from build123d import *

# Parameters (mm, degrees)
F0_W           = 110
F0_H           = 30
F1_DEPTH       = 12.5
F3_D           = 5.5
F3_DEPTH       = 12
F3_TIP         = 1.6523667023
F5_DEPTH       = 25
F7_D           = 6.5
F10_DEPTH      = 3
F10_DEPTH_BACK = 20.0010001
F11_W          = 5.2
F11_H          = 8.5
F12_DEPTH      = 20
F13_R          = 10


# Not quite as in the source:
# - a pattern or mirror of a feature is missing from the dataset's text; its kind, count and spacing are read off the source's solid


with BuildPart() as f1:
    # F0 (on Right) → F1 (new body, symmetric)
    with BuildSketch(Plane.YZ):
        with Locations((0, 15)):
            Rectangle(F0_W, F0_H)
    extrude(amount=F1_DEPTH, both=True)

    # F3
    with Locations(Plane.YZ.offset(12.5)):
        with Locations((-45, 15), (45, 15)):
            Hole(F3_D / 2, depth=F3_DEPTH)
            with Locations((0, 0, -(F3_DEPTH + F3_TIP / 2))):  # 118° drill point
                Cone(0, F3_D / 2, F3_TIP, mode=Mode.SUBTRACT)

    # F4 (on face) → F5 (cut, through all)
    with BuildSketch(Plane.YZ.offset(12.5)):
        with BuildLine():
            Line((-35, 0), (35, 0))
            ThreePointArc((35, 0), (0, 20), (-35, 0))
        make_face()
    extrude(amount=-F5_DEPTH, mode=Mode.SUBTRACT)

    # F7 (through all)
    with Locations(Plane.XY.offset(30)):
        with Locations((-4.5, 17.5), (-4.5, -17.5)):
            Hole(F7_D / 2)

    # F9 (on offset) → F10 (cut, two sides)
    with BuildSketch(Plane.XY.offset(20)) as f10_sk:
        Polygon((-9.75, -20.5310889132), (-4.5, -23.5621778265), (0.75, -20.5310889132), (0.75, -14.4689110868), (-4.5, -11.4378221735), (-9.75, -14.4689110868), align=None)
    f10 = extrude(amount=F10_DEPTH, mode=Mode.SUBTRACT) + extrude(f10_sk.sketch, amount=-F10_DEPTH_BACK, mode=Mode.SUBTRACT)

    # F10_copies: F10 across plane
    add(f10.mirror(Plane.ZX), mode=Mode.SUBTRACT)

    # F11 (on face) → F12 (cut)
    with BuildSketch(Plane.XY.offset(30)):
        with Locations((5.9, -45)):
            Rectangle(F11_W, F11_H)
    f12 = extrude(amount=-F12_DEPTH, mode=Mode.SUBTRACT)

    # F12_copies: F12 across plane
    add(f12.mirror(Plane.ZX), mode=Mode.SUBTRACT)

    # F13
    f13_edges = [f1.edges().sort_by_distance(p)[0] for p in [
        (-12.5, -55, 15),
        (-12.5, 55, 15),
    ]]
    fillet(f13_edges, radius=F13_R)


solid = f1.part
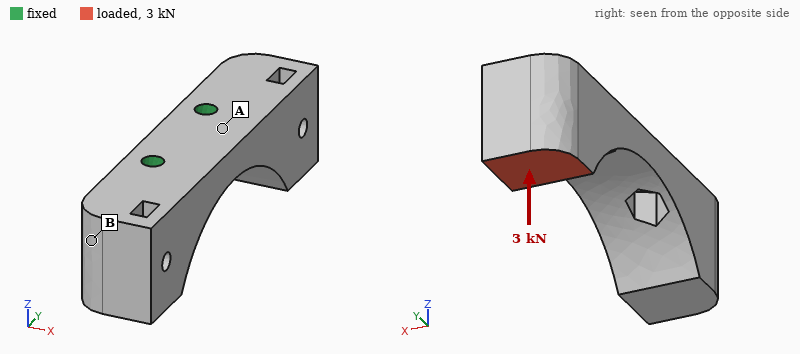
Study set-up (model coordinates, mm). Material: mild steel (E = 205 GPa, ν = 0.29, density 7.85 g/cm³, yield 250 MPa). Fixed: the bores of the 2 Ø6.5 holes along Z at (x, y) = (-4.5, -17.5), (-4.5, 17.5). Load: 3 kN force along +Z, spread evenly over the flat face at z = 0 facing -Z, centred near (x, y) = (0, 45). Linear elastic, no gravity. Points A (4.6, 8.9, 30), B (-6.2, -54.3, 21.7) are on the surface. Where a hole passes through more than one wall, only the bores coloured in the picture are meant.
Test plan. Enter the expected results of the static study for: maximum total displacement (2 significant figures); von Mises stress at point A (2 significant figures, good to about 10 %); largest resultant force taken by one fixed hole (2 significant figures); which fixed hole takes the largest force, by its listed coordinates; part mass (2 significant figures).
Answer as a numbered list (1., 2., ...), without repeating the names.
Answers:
1. 70 µm
2. 47 MPa
3. 4.5 kN
4. (-4.5, 17.5)
5. 410 g
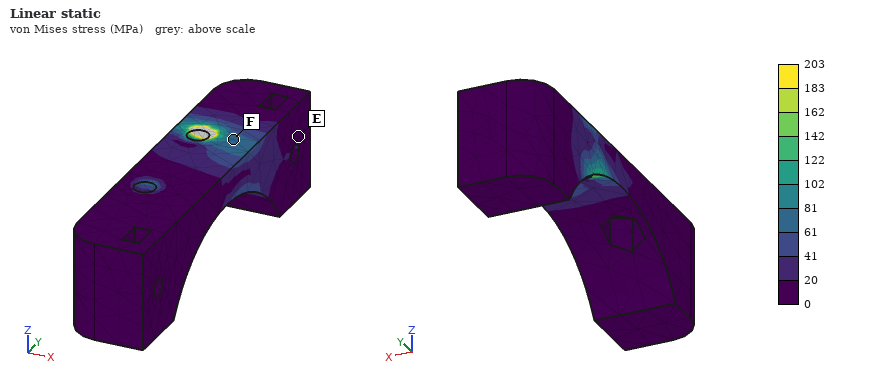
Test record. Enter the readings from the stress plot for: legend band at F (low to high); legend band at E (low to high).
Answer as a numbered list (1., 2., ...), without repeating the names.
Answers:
1. 61 to 81 MPa
2. 0 to 20 MPa
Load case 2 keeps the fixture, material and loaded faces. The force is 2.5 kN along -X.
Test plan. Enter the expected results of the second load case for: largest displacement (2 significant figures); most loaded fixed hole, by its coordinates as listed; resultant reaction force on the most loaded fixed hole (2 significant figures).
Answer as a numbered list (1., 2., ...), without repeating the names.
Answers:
1. 60 µm
2. (-4.5, 17.5)
3. 3.9 kN
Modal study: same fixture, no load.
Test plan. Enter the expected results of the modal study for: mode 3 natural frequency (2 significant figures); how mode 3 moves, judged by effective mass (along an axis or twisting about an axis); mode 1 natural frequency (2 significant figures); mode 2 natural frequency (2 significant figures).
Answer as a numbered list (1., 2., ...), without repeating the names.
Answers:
1. 4800 Hz
2. along X
3. 3400 Hz
4. 3600 Hz
